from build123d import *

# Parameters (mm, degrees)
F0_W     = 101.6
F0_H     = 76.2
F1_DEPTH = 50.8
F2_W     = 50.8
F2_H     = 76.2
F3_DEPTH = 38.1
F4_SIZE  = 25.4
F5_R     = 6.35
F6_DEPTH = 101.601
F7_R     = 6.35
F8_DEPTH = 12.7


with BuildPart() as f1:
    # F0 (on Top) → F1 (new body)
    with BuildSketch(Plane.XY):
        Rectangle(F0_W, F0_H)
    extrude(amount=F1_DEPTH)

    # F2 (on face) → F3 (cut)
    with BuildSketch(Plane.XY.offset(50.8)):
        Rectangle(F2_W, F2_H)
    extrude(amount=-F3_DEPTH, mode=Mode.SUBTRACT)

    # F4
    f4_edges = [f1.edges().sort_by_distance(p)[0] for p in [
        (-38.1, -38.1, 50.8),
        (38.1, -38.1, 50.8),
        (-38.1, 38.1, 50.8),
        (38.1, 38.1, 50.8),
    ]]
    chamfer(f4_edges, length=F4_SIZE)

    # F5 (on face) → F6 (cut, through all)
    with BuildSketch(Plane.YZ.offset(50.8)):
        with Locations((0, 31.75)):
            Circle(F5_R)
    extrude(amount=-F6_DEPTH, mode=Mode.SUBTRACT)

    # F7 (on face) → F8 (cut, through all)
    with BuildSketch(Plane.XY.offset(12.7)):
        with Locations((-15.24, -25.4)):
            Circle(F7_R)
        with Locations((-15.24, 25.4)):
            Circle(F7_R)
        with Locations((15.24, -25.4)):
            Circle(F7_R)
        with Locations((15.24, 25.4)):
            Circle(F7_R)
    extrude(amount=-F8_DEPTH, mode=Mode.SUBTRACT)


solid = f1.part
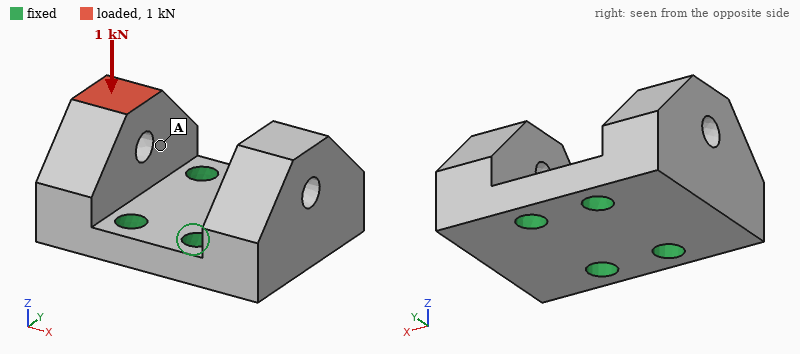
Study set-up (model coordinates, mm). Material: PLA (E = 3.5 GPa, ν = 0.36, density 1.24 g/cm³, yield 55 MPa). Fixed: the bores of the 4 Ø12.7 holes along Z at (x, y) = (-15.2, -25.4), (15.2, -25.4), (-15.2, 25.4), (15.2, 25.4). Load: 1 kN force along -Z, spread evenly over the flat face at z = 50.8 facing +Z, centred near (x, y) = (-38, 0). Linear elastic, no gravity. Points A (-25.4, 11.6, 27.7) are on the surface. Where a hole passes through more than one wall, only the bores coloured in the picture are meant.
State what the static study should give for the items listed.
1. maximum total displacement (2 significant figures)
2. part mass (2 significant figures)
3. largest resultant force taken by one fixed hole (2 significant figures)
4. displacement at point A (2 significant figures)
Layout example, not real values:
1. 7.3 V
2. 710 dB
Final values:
1. 0.24 mm
2. 250 g
3. 550 N
4. 0.091 mm
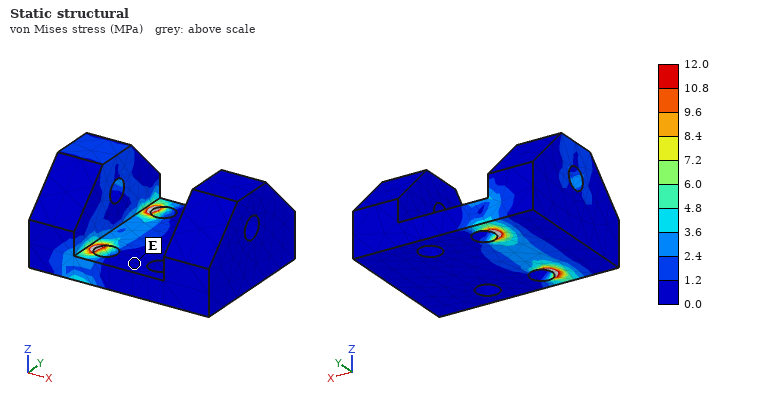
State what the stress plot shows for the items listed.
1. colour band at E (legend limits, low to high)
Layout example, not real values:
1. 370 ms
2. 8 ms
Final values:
1. 0.0 to 1.2 MPa
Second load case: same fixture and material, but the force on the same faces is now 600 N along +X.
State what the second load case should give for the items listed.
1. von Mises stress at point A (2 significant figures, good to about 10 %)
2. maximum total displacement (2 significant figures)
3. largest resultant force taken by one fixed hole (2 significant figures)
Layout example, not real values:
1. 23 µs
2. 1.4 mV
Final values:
1. 3.5 MPa
2. 0.48 mm
3. 280 N
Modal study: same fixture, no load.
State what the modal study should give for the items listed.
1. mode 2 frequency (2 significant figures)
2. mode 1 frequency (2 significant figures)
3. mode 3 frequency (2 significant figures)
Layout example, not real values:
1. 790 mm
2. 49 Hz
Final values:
1. 1100 Hz
2. 1100 Hz
3. 2600 Hz
